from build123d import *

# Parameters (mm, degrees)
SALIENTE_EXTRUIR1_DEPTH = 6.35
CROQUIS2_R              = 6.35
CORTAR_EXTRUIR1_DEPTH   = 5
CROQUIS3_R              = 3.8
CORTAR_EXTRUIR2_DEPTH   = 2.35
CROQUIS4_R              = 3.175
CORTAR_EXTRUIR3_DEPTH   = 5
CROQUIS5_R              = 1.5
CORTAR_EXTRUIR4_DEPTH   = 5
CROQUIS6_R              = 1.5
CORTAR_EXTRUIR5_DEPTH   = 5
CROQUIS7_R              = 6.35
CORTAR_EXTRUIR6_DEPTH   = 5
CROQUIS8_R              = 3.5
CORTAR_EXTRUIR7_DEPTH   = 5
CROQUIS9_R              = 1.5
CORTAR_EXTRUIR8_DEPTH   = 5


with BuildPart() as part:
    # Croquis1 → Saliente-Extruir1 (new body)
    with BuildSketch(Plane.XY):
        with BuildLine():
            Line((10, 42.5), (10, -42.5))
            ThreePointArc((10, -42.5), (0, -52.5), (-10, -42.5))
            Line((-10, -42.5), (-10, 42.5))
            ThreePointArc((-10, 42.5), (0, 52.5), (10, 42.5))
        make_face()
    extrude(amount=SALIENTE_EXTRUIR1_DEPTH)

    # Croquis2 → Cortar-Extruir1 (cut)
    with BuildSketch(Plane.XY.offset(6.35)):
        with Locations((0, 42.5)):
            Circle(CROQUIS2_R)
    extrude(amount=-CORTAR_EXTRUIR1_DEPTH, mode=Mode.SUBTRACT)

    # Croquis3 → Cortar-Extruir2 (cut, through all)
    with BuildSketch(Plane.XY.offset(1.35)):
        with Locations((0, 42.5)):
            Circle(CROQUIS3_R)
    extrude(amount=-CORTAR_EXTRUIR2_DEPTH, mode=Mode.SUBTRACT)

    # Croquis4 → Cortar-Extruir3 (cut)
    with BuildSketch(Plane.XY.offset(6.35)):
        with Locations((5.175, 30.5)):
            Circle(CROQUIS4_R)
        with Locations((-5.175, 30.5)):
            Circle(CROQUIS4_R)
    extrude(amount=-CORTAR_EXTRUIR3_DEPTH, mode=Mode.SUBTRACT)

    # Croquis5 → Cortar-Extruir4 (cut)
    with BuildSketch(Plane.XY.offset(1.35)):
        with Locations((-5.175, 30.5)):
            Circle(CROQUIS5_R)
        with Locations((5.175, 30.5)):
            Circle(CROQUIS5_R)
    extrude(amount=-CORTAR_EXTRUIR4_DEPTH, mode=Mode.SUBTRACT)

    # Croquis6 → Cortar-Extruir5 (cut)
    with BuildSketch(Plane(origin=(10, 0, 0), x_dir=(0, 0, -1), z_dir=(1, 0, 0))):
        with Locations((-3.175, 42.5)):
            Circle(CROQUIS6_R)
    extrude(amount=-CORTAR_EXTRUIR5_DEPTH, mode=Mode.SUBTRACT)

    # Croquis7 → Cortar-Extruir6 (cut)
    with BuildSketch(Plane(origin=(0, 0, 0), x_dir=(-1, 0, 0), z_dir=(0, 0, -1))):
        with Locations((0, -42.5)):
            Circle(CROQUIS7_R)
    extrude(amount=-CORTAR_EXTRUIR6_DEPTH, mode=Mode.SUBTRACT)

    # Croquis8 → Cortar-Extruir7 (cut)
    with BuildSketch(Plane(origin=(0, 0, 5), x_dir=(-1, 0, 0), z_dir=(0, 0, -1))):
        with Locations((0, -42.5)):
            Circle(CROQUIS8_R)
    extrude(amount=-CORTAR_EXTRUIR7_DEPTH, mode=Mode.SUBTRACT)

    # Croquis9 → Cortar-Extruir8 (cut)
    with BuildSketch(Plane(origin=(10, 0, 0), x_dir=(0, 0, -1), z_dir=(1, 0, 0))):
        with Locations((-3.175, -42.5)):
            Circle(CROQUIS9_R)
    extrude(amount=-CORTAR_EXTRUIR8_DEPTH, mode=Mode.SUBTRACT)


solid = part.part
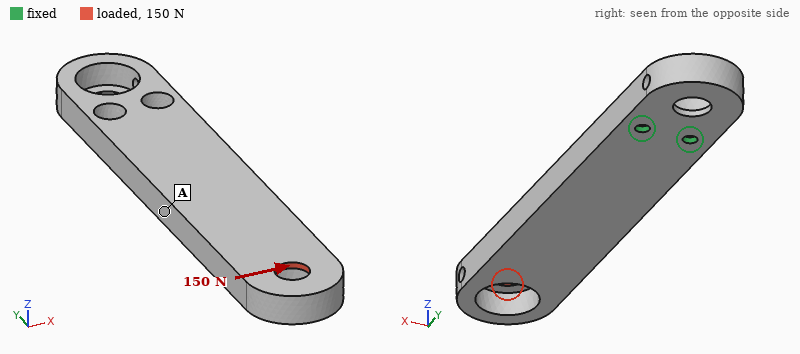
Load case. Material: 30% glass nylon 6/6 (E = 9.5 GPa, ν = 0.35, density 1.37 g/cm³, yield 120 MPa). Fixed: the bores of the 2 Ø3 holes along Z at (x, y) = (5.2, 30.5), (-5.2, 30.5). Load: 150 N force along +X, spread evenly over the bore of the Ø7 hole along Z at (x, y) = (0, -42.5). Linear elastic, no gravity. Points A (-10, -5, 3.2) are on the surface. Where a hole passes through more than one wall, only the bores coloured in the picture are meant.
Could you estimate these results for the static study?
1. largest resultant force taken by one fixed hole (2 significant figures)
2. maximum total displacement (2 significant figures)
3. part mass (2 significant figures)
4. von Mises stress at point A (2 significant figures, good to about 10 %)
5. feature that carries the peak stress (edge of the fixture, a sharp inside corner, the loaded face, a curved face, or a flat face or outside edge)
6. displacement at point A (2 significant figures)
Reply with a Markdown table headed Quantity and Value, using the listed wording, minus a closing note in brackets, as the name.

| Quantity | Value |
|---|---|
| largest resultant force taken by one fixed hole | 920 N |
| maximum total displacement | 1.0 mm |
| part mass | 15 g |
| von Mises stress at point A | 14 MPa |
| feature that carries the peak stress | edge of the fixture |
| displacement at point A | 0.35 mm |
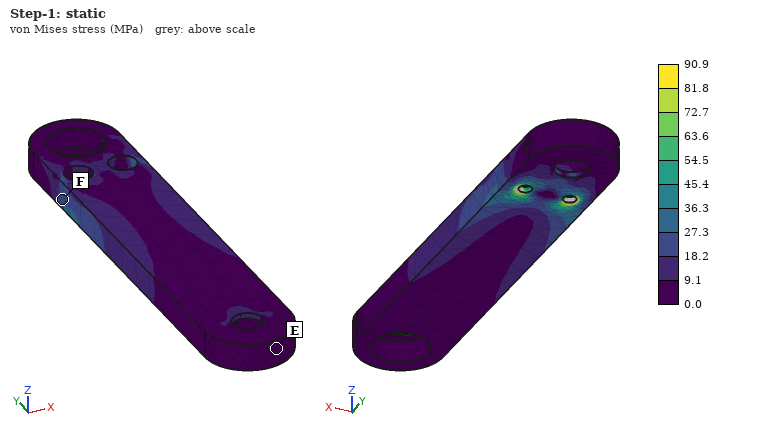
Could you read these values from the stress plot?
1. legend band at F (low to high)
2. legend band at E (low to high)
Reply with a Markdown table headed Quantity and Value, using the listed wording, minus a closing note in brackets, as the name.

| Quantity | Value |
|---|---|
| legend band at F | 18.2 to 27.3 MPa |
| legend band at E | 0.0 to 9.1 MPa |
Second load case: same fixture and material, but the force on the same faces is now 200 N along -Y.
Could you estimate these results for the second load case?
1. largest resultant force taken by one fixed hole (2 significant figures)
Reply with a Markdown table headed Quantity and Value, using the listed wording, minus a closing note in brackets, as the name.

| Quantity | Value |
|---|---|
| largest resultant force taken by one fixed hole | 100 N |
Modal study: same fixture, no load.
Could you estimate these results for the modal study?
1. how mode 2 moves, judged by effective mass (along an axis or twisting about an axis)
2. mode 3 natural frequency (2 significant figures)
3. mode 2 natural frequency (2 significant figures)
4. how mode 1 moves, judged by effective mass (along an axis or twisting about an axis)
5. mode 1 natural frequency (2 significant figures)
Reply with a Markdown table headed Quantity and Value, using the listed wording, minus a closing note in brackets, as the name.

| Quantity | Value |
|---|---|
| how mode 2 moves, judged by effective mass | along X |
| mode 3 natural frequency | 2000 Hz |
| mode 2 natural frequency | 1000 Hz |
| how mode 1 moves, judged by effective mass | along Z |
| mode 1 natural frequency | 260 Hz |
